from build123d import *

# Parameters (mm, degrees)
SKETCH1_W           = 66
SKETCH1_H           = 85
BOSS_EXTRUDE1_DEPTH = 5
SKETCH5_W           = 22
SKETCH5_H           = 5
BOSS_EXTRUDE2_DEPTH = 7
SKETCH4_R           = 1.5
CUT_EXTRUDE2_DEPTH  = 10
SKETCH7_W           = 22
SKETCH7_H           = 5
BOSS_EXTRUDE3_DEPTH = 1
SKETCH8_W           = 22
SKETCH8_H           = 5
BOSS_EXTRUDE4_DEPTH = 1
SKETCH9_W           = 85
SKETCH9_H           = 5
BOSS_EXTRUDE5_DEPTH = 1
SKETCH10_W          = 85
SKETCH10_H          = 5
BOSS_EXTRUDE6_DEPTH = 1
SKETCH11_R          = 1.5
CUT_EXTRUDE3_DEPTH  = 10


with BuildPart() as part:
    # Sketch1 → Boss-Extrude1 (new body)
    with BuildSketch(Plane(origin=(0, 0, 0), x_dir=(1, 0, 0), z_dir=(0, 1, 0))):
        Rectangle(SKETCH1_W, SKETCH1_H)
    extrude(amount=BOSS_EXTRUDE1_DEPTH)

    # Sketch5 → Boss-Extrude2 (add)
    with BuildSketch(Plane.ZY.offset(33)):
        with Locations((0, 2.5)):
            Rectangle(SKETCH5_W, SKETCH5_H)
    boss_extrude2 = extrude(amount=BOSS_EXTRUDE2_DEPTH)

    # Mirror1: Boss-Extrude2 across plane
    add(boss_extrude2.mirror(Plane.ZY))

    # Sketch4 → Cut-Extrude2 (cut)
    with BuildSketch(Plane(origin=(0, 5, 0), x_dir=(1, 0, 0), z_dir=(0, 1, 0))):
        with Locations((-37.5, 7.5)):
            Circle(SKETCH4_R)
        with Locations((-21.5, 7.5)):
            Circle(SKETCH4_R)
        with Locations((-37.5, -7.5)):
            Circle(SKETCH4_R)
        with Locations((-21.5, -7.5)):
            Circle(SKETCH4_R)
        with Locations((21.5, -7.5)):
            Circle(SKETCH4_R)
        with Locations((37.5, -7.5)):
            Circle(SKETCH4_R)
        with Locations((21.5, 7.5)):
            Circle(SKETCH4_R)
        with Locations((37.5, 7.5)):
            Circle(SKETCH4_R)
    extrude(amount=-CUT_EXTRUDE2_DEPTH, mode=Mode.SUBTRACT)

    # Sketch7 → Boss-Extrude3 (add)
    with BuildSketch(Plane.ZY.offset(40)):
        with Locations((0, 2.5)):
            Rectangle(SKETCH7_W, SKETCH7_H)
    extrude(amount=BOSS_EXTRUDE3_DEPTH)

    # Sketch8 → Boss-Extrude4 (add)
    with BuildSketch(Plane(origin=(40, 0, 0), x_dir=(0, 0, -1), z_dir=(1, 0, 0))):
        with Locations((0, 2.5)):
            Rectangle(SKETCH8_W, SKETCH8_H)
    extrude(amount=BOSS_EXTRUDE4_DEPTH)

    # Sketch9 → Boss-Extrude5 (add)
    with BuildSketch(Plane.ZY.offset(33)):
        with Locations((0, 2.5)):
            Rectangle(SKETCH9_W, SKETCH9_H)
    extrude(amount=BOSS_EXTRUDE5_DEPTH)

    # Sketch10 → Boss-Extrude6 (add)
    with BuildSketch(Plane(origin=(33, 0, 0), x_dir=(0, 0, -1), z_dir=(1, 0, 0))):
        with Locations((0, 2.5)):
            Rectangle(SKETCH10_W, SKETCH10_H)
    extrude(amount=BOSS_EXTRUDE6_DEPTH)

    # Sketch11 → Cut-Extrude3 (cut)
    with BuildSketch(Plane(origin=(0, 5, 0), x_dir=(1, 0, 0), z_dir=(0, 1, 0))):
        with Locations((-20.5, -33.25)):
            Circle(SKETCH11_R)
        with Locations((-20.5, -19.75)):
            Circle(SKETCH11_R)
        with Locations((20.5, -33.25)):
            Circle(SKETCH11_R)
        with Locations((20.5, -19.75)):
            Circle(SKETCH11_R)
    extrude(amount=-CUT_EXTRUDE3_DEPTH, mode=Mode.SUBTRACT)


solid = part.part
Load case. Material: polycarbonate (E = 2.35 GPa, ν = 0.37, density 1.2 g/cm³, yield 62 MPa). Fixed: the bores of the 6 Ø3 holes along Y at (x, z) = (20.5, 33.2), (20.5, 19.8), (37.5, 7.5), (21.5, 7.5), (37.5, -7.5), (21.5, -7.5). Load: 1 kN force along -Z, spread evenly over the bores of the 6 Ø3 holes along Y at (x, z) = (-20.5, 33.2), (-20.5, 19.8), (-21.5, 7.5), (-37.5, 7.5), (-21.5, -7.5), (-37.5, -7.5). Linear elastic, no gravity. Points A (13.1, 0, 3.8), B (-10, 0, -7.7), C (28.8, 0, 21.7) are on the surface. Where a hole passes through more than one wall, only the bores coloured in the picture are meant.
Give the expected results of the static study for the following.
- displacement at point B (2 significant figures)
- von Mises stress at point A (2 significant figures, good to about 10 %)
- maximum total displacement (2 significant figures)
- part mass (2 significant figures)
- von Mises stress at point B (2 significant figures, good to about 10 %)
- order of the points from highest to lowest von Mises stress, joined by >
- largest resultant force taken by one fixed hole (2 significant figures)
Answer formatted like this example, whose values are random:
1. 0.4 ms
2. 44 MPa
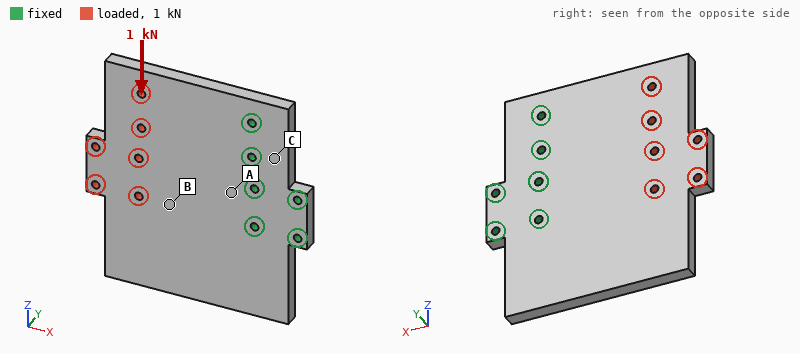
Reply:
1. 0.28 mm
2. 9.0 MPa
3. 0.55 mm
4. 36 g
5. 5.1 MPa
6. A > B > C
7. 990 N
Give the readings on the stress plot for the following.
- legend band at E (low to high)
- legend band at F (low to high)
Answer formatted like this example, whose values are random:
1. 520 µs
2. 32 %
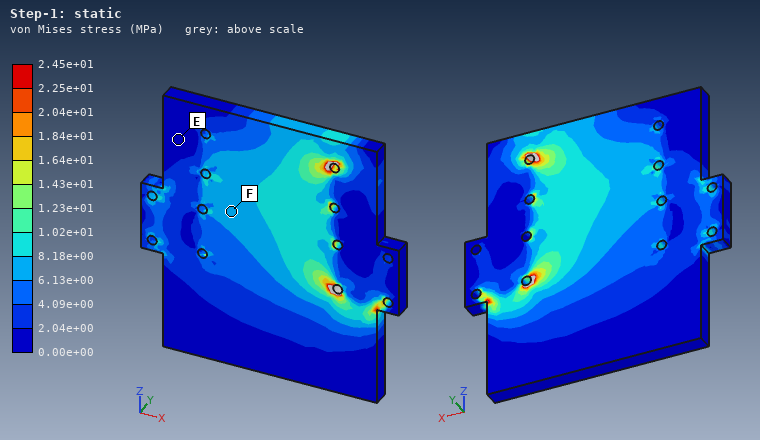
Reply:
1. 0.00e+00 to 2.04e+00 MPa
2. 6.13e+00 to 8.18e+00 MPa
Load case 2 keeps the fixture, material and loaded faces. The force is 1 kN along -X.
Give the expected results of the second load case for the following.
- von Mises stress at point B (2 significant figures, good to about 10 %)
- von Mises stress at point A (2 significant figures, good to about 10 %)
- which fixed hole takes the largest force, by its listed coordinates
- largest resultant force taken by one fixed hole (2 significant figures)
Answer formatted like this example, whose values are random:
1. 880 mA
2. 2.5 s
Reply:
1. 3.7 MPa
2. 3.4 MPa
3. (21.5, -7.5)
4. 320 N
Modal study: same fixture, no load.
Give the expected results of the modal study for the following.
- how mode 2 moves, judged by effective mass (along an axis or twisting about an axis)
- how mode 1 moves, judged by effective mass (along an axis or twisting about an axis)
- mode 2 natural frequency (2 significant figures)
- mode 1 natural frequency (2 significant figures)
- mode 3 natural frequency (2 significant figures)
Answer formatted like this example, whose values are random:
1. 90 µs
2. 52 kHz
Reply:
1. twisting about X
2. along Y
3. 530 Hz
4. 320 Hz
5. 990 Hz
